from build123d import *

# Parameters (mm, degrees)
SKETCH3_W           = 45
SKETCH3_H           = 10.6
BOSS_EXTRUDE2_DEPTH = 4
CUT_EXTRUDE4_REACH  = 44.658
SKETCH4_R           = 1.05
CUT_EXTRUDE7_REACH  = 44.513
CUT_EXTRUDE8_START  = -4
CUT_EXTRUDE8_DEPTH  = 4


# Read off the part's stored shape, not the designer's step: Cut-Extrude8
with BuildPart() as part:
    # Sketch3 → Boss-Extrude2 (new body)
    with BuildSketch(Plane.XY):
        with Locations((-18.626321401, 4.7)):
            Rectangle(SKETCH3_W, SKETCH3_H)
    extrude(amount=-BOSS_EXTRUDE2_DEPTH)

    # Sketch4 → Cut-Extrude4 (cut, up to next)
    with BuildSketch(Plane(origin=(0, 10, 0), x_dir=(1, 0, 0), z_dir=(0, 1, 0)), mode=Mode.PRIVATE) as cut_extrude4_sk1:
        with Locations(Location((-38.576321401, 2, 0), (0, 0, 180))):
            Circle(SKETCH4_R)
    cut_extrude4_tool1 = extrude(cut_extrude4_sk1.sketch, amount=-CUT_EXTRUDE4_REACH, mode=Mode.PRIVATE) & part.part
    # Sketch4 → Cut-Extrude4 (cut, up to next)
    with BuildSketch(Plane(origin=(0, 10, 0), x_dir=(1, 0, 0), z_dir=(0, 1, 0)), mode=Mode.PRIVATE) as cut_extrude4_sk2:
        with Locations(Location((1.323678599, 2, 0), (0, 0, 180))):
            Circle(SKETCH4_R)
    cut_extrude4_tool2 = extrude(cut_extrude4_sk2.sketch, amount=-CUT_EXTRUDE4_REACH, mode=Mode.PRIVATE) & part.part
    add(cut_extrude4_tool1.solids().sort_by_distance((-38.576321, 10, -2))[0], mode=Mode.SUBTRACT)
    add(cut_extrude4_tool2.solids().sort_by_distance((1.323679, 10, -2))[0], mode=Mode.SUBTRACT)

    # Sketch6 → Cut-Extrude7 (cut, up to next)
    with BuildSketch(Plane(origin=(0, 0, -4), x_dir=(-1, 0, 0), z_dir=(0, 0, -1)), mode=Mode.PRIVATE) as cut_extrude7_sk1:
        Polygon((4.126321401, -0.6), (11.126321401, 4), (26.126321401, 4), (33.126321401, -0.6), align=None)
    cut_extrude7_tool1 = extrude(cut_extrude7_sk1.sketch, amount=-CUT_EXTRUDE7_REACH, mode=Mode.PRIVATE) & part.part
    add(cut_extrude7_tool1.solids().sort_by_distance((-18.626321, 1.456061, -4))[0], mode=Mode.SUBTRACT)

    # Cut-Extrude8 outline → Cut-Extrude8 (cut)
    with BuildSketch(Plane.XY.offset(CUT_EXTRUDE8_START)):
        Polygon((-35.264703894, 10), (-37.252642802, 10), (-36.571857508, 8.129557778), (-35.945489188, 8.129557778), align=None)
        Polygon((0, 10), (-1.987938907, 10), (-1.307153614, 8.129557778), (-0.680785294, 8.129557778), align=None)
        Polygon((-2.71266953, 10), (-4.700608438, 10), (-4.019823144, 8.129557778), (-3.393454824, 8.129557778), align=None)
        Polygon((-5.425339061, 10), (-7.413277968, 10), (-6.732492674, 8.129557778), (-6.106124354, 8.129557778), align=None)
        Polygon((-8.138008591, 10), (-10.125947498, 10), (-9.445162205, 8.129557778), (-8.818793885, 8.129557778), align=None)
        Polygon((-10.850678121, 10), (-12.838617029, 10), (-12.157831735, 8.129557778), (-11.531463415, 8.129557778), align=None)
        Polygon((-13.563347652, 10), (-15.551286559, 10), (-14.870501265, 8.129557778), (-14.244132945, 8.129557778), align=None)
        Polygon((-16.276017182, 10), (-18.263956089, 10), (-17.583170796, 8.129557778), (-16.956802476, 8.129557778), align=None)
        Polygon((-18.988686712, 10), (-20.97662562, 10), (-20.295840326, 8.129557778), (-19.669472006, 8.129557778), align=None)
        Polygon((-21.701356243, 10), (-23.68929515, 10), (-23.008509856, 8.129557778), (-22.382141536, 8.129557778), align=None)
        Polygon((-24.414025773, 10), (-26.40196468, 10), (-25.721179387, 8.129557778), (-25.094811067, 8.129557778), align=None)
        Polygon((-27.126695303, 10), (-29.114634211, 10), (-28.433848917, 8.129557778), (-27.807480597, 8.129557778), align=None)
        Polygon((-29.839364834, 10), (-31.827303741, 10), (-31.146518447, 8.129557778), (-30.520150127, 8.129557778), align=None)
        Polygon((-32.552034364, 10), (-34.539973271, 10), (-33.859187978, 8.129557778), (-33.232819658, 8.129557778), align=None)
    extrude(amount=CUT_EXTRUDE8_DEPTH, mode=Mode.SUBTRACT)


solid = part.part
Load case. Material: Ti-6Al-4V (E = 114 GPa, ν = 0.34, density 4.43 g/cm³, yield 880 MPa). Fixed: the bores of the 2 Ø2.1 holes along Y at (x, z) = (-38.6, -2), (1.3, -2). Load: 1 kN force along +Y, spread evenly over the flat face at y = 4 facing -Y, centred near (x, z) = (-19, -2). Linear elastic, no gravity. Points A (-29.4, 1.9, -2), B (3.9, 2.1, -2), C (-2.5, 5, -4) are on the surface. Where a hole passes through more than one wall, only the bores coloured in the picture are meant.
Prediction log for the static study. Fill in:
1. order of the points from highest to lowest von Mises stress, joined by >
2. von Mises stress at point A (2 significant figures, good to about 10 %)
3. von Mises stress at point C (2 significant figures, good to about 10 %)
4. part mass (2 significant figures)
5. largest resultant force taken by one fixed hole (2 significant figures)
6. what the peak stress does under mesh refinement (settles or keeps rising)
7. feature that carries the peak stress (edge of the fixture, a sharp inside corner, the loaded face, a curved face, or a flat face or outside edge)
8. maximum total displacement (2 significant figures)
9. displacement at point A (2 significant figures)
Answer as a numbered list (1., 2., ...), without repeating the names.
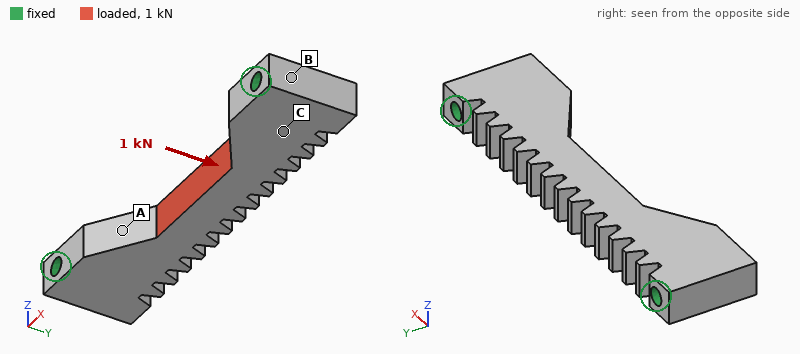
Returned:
1. A > C > B
2. 93 MPa
3. 28 MPa
4. 5.7 g
5. 620 N
6. keeps rising
7. edge of the fixture
8. 30 µm
9. 9.7 µm
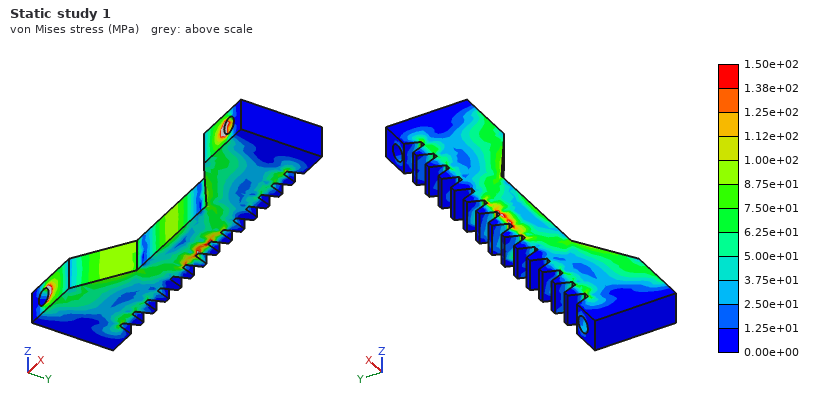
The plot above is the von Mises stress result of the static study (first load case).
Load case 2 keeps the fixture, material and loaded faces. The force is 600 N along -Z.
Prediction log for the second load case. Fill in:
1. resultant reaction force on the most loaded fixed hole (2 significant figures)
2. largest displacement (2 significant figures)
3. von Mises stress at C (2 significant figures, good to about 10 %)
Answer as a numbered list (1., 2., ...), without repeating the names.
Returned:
1. 300 N
2. 56 µm
3. 90 MPa
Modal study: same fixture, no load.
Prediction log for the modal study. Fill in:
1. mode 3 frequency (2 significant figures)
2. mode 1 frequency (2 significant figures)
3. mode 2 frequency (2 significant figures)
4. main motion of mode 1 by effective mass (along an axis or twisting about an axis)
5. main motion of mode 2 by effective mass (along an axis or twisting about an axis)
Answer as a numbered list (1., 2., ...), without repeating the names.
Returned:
1. 30 kHz
2. 13 kHz
3. 24 kHz
4. along Z
5. along Y
